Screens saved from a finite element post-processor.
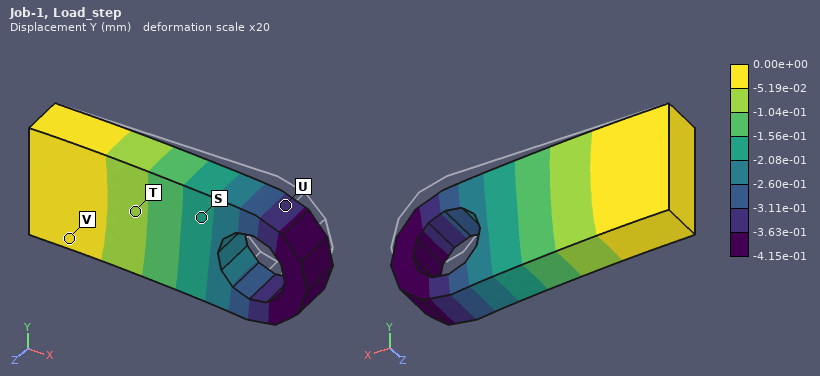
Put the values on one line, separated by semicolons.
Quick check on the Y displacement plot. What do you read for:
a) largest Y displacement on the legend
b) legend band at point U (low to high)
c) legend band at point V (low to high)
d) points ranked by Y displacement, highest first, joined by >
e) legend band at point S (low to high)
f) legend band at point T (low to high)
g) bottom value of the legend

0.00e+00 mm; -3.63e-01 to -3.11e-01 mm; -5.19e-02 to 0.00e+00 mm; V > T > S > U; -2.08e-01 to -1.56e-01 mm; -1.04e-01 to -5.19e-02 mm; -4.15e-01 mm
